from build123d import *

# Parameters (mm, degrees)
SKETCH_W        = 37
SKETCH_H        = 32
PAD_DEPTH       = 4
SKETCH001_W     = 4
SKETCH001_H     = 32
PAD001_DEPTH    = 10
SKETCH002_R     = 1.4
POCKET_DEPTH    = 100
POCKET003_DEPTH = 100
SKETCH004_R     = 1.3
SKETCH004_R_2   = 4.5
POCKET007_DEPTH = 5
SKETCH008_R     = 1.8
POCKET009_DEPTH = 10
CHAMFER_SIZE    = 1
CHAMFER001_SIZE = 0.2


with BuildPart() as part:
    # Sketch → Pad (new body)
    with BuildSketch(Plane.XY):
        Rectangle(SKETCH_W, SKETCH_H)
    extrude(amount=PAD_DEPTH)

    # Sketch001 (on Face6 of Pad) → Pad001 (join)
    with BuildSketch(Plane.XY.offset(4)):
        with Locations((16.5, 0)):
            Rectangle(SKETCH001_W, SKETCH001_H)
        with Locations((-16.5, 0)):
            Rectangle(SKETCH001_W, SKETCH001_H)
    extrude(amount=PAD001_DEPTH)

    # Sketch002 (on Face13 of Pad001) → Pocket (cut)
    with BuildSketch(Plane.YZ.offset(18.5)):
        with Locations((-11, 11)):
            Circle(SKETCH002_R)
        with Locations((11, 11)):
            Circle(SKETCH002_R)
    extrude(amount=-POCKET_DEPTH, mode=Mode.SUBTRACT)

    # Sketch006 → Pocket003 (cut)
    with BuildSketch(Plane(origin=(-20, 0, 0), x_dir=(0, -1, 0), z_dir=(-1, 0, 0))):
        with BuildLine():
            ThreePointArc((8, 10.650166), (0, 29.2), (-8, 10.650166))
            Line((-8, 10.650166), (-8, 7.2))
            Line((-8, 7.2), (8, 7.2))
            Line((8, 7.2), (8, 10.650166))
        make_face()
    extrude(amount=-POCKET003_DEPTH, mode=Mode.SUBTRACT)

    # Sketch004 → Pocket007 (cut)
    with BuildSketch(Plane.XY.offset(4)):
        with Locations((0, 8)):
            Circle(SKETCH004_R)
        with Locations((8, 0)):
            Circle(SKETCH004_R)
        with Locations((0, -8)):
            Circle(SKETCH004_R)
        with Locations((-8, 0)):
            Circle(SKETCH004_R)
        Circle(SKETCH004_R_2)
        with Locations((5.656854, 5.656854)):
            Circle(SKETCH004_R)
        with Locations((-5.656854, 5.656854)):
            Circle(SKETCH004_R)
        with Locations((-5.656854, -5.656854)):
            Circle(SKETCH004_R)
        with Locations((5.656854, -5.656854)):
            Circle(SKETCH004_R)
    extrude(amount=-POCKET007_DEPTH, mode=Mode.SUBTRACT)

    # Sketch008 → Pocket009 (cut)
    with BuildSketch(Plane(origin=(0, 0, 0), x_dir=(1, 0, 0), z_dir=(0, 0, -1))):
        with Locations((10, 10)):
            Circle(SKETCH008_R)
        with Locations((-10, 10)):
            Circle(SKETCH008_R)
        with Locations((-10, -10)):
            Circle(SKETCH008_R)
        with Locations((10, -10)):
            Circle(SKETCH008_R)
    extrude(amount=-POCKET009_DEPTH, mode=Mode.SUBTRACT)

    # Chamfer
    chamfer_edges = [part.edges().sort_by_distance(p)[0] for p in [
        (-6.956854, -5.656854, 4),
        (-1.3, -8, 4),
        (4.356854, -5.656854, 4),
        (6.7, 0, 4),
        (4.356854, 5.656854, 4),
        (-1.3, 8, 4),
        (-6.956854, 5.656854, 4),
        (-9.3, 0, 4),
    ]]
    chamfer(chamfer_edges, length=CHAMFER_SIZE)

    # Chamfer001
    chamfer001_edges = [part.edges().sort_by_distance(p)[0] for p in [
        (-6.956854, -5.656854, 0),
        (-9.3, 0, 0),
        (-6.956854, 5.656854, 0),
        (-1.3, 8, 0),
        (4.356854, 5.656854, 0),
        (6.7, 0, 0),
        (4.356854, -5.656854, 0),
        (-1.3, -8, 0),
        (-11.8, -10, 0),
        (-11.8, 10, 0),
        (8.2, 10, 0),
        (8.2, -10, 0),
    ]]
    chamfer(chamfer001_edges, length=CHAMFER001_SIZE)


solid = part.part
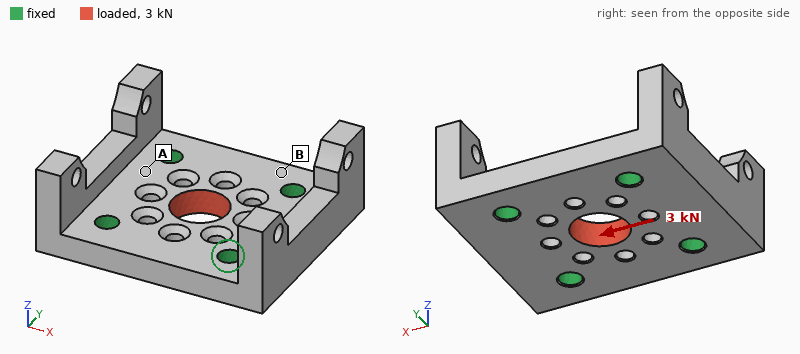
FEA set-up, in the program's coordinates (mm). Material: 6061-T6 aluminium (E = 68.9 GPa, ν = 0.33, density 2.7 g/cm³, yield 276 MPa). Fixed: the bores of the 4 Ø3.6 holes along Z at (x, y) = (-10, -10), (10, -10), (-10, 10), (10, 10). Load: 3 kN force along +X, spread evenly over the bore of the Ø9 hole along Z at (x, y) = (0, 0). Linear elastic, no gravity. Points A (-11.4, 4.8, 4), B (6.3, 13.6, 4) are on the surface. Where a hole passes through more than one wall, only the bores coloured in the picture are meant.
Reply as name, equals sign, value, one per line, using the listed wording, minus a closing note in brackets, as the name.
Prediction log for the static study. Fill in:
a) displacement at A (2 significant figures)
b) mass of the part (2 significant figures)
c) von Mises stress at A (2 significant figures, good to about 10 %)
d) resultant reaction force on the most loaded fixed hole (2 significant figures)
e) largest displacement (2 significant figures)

displacement at A = 2.2 µm
mass of the part = 15 g
von Mises stress at A = 19 MPa
resultant reaction force on the most loaded fixed hole = 770 N
largest displacement = 6.2 µm
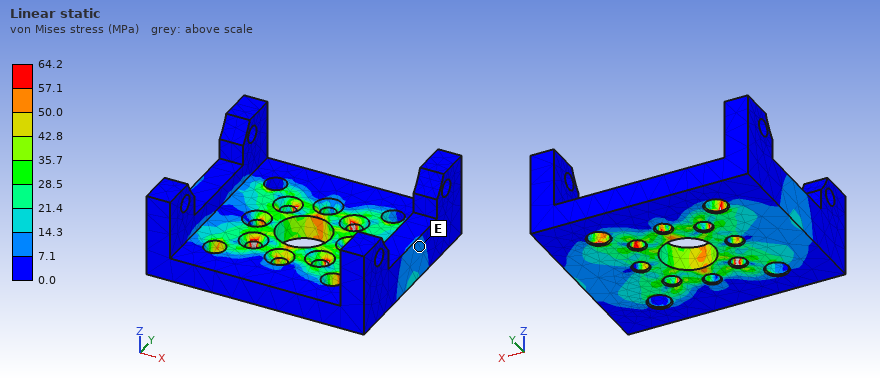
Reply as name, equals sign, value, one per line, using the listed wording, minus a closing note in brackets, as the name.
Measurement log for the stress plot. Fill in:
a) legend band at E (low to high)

legend band at E = 7.1 to 14.3 MPa
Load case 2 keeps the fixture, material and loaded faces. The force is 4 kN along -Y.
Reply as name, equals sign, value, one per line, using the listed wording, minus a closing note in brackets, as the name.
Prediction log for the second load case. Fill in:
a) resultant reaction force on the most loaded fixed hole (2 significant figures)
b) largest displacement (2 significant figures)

resultant reaction force on the most loaded fixed hole = 1.1 kN
largest displacement = 8.8 µm
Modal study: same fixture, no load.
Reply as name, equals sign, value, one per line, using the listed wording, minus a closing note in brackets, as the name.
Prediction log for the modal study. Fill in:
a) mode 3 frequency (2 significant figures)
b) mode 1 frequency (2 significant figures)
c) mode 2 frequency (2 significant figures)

mode 3 frequency = 18 kHz
mode 1 frequency = 16 kHz
mode 2 frequency = 16 kHz
